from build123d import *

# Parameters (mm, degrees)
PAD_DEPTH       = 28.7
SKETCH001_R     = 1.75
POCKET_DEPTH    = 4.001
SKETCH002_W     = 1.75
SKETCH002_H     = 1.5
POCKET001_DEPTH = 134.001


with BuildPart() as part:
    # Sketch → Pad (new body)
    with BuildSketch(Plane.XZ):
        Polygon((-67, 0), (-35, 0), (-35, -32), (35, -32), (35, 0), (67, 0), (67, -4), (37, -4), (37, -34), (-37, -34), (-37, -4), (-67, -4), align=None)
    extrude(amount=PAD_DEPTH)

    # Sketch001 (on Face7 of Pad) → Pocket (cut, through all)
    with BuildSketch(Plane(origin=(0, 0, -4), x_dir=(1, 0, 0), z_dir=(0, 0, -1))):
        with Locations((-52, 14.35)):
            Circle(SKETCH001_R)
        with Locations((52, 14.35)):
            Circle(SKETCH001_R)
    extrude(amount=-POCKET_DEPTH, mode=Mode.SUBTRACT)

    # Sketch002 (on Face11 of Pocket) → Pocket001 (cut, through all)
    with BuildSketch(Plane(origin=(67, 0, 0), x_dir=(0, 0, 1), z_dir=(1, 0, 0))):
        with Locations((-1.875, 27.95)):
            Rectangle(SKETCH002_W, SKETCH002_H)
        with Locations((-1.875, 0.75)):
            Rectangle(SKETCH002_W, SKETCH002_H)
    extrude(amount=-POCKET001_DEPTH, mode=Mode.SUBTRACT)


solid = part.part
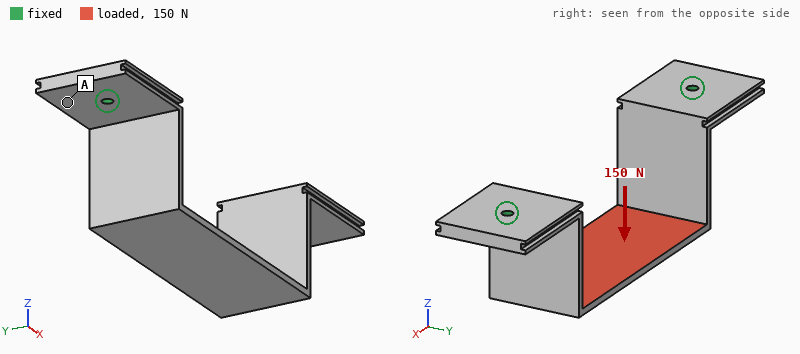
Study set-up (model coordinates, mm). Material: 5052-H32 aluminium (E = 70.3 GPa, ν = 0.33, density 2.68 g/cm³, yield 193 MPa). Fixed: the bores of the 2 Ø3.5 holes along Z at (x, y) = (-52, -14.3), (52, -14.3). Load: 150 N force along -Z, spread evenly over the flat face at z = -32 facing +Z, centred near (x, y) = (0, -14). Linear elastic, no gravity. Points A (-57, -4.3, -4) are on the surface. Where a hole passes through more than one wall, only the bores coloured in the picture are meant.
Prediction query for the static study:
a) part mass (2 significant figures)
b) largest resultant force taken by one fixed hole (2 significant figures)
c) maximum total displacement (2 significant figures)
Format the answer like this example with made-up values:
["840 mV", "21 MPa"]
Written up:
["39 g", "86 N", "0.18 mm"]
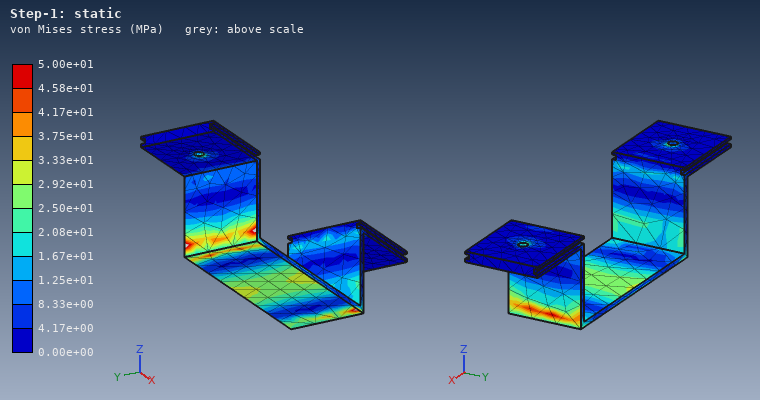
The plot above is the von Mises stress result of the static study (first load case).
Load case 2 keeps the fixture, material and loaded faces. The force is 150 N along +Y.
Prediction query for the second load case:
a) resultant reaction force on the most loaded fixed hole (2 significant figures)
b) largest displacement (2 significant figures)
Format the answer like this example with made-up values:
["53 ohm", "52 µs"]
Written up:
["75 N", "0.10 mm"]
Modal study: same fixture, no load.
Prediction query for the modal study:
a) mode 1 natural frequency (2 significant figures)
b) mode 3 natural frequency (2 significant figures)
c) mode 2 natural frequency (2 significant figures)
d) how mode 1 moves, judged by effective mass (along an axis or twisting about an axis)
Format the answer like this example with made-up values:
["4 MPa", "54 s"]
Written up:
["1000 Hz", "1600 Hz", "1600 Hz", "along X"]
